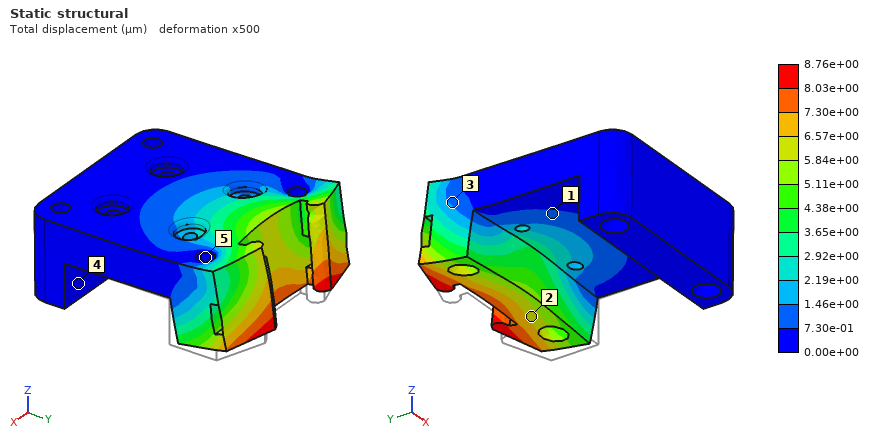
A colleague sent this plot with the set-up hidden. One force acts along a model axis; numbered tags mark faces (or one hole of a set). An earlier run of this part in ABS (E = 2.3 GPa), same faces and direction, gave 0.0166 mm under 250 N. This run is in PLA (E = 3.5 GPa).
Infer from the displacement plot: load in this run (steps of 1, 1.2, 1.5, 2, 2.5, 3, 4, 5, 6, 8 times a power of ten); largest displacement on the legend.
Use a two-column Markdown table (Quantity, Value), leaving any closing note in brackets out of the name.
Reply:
| Quantity | Value |
|---|---|
| load in this run | 200 N |
| largest displacement on the legend | 8.76e+00 µm |
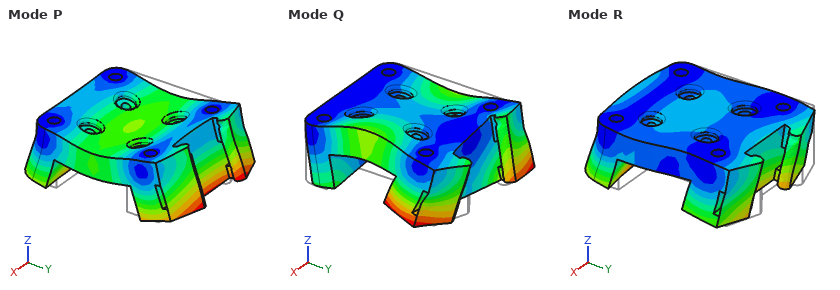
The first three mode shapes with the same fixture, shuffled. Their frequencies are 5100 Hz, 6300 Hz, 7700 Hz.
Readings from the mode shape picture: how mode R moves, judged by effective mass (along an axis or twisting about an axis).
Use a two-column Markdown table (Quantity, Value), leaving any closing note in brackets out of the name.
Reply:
| Quantity | Value |
|---|---|
| how mode R moves, judged by effective mass | along Y |
